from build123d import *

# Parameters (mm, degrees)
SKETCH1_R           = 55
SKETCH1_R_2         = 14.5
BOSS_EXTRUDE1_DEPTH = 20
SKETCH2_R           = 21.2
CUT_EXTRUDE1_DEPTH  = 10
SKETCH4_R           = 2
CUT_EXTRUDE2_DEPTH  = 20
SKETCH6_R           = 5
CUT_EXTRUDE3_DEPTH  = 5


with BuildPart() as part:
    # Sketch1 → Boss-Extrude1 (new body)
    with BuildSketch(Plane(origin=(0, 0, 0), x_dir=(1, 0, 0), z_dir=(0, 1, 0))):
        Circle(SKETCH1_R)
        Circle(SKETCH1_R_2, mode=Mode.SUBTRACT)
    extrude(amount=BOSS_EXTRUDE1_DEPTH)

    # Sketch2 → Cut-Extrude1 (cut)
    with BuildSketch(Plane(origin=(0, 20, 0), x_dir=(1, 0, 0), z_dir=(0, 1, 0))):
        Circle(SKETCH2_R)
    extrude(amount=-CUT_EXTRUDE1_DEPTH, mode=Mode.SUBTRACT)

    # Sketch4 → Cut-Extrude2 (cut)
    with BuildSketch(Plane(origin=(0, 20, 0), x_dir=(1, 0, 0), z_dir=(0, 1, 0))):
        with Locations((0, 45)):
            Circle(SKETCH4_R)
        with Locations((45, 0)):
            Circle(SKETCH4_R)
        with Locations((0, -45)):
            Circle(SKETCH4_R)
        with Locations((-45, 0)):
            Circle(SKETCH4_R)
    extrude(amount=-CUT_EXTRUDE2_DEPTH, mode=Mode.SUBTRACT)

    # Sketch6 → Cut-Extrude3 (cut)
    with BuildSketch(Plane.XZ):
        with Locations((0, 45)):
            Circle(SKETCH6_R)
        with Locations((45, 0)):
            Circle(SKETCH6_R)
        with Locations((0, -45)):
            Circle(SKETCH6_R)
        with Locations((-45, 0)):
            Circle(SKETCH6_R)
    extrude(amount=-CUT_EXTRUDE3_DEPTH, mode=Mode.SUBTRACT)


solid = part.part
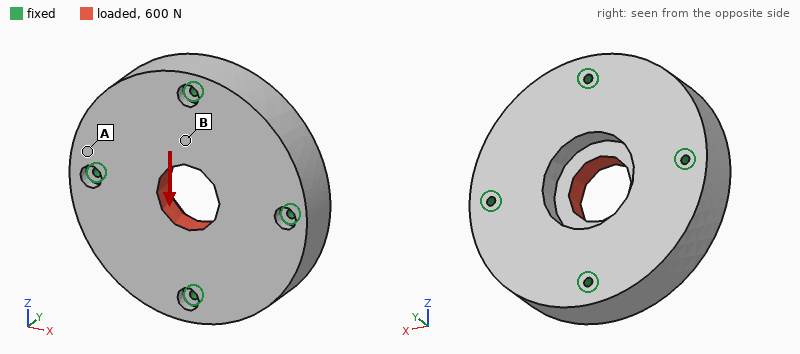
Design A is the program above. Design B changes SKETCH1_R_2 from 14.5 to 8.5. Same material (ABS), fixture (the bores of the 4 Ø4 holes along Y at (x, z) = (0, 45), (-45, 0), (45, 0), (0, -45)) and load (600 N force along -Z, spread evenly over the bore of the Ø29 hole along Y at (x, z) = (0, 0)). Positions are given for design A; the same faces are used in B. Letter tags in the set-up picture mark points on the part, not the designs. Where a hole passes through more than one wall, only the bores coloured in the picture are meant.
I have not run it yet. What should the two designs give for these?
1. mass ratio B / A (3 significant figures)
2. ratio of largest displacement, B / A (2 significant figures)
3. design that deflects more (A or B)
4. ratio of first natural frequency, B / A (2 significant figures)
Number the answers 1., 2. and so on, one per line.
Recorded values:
1. 1.03
2. 1.2
3. B
4. 1.0
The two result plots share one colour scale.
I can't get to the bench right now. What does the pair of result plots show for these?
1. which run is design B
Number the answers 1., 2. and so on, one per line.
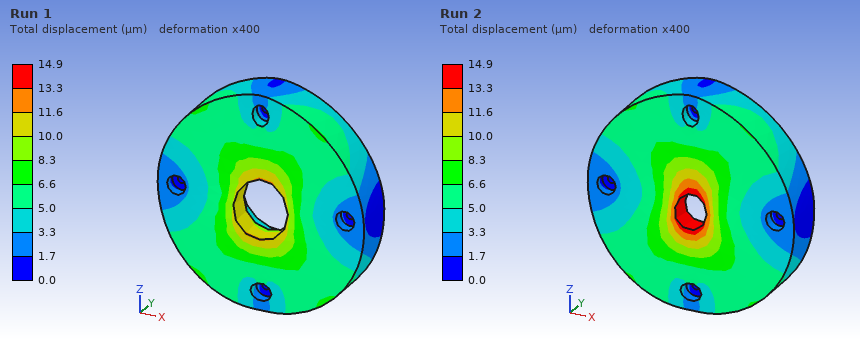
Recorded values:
1. Run 2
